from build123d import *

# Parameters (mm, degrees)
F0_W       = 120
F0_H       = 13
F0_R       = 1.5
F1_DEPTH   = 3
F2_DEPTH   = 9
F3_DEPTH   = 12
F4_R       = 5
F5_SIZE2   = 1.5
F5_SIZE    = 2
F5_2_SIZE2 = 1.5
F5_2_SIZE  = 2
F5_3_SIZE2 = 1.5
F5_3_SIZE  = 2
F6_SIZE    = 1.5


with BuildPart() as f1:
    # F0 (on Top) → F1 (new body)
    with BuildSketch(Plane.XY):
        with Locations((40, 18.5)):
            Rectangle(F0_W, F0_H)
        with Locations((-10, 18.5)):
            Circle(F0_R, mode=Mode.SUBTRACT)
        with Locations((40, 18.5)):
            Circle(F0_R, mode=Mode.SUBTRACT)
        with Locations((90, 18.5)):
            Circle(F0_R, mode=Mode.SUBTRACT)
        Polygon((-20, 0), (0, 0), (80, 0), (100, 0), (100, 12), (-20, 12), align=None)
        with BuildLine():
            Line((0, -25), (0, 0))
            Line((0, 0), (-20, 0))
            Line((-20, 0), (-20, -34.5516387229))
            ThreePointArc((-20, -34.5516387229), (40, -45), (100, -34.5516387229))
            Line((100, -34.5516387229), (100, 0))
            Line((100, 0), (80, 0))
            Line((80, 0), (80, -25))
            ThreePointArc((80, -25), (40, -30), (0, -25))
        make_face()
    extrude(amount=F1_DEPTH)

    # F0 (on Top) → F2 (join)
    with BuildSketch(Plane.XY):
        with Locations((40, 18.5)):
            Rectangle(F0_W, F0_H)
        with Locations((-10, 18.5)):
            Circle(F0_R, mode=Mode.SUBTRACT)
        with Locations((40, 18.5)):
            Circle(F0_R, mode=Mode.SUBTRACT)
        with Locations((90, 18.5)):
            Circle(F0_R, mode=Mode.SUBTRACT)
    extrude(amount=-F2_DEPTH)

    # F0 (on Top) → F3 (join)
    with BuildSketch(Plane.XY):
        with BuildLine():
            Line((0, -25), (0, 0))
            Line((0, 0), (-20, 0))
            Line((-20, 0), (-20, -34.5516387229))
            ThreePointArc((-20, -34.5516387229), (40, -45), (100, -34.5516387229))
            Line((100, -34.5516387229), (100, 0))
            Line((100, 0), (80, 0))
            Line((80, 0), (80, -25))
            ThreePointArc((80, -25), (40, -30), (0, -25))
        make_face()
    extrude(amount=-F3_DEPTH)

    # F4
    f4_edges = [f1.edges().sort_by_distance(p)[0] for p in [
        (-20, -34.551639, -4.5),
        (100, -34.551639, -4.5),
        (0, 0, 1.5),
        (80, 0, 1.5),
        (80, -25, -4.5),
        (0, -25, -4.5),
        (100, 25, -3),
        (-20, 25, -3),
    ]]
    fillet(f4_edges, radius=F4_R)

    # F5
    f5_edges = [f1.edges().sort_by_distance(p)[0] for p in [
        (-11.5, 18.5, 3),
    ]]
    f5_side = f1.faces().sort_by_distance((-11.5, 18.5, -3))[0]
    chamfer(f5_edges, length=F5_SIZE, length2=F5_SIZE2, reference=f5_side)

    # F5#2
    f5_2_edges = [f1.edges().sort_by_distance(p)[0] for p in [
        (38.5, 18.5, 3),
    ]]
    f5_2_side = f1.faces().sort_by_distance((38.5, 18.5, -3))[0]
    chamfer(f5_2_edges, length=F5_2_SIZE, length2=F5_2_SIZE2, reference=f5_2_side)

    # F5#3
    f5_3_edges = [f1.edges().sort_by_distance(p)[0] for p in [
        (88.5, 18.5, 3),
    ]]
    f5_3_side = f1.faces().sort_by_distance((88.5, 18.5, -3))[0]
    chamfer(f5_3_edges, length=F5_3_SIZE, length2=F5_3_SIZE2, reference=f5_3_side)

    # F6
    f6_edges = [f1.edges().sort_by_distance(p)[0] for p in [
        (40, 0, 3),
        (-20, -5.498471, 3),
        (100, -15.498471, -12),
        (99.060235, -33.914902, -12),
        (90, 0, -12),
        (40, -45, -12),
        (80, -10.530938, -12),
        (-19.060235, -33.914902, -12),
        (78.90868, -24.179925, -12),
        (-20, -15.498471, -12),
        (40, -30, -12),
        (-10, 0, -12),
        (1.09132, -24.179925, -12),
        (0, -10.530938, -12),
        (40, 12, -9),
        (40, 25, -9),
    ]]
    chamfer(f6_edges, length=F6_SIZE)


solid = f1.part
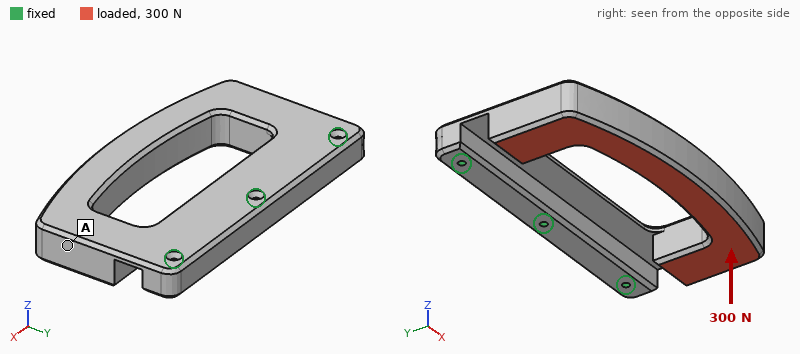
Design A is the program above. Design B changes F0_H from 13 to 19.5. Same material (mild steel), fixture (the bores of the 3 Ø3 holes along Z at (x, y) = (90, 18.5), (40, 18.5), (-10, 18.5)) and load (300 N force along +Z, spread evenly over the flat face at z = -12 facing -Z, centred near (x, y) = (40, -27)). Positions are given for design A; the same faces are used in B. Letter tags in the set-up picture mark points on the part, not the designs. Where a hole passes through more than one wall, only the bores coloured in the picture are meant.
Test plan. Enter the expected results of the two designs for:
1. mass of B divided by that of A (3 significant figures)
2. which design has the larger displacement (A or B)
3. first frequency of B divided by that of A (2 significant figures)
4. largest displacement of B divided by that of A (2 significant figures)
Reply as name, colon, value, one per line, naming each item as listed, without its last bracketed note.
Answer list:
mass of B divided by that of A: 1.13
which design has the larger displacement: A
first frequency of B divided by that of A: 1.1
largest displacement of B divided by that of A: 0.77
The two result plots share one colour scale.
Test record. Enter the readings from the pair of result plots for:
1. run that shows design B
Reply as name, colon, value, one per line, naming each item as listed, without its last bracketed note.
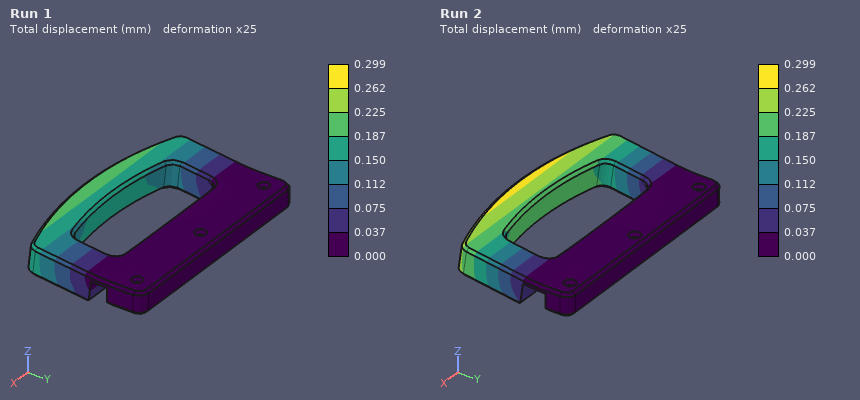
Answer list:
run that shows design B: Run 1
